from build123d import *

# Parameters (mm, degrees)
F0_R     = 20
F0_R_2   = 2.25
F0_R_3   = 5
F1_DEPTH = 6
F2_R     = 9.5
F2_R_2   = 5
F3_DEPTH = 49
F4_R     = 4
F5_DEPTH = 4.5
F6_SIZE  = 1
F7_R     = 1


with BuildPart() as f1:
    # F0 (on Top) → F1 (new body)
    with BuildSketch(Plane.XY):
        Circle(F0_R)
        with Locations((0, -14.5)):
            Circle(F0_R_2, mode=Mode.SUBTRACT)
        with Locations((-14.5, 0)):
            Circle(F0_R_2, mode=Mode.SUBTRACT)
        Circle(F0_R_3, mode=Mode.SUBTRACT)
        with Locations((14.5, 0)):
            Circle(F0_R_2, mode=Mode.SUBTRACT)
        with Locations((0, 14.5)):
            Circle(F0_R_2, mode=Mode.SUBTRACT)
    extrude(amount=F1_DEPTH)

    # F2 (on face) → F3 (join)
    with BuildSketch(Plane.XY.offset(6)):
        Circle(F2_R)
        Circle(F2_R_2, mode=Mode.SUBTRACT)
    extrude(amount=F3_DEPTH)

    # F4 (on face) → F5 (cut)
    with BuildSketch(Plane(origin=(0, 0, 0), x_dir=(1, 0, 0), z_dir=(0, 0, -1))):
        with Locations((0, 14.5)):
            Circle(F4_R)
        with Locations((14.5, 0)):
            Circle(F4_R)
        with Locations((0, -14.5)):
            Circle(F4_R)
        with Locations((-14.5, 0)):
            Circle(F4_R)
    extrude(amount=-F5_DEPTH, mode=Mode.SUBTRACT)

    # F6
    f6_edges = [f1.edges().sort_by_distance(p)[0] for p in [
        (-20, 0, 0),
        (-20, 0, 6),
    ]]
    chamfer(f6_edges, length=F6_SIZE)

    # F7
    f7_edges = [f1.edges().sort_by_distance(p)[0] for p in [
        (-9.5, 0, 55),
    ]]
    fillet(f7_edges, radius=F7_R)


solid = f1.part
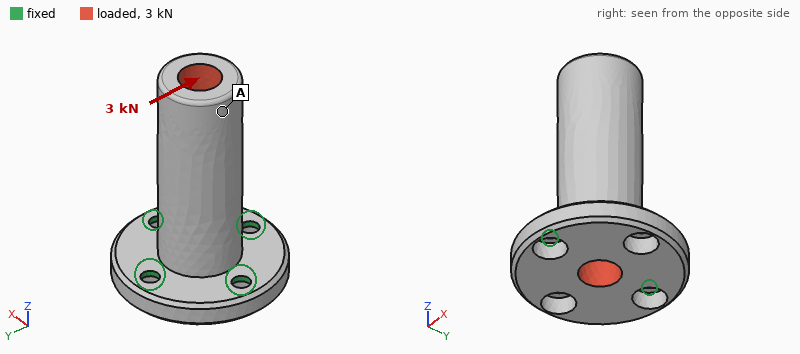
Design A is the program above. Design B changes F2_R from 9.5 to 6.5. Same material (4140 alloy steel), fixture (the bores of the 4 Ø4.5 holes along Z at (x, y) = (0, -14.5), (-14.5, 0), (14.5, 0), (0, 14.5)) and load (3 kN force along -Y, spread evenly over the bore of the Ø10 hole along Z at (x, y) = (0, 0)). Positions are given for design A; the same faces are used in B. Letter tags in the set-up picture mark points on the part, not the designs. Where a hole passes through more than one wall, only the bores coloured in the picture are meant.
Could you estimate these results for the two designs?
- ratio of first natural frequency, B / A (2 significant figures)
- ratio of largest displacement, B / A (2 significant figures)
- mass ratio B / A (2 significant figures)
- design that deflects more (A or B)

0.95
4.2
0.54
B
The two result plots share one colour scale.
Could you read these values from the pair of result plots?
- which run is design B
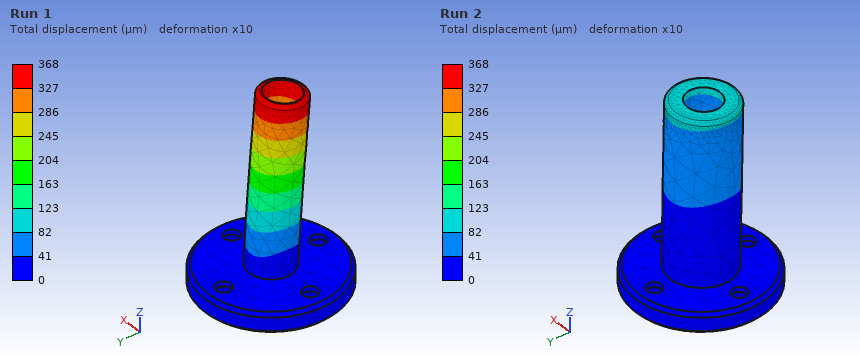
Run 1
